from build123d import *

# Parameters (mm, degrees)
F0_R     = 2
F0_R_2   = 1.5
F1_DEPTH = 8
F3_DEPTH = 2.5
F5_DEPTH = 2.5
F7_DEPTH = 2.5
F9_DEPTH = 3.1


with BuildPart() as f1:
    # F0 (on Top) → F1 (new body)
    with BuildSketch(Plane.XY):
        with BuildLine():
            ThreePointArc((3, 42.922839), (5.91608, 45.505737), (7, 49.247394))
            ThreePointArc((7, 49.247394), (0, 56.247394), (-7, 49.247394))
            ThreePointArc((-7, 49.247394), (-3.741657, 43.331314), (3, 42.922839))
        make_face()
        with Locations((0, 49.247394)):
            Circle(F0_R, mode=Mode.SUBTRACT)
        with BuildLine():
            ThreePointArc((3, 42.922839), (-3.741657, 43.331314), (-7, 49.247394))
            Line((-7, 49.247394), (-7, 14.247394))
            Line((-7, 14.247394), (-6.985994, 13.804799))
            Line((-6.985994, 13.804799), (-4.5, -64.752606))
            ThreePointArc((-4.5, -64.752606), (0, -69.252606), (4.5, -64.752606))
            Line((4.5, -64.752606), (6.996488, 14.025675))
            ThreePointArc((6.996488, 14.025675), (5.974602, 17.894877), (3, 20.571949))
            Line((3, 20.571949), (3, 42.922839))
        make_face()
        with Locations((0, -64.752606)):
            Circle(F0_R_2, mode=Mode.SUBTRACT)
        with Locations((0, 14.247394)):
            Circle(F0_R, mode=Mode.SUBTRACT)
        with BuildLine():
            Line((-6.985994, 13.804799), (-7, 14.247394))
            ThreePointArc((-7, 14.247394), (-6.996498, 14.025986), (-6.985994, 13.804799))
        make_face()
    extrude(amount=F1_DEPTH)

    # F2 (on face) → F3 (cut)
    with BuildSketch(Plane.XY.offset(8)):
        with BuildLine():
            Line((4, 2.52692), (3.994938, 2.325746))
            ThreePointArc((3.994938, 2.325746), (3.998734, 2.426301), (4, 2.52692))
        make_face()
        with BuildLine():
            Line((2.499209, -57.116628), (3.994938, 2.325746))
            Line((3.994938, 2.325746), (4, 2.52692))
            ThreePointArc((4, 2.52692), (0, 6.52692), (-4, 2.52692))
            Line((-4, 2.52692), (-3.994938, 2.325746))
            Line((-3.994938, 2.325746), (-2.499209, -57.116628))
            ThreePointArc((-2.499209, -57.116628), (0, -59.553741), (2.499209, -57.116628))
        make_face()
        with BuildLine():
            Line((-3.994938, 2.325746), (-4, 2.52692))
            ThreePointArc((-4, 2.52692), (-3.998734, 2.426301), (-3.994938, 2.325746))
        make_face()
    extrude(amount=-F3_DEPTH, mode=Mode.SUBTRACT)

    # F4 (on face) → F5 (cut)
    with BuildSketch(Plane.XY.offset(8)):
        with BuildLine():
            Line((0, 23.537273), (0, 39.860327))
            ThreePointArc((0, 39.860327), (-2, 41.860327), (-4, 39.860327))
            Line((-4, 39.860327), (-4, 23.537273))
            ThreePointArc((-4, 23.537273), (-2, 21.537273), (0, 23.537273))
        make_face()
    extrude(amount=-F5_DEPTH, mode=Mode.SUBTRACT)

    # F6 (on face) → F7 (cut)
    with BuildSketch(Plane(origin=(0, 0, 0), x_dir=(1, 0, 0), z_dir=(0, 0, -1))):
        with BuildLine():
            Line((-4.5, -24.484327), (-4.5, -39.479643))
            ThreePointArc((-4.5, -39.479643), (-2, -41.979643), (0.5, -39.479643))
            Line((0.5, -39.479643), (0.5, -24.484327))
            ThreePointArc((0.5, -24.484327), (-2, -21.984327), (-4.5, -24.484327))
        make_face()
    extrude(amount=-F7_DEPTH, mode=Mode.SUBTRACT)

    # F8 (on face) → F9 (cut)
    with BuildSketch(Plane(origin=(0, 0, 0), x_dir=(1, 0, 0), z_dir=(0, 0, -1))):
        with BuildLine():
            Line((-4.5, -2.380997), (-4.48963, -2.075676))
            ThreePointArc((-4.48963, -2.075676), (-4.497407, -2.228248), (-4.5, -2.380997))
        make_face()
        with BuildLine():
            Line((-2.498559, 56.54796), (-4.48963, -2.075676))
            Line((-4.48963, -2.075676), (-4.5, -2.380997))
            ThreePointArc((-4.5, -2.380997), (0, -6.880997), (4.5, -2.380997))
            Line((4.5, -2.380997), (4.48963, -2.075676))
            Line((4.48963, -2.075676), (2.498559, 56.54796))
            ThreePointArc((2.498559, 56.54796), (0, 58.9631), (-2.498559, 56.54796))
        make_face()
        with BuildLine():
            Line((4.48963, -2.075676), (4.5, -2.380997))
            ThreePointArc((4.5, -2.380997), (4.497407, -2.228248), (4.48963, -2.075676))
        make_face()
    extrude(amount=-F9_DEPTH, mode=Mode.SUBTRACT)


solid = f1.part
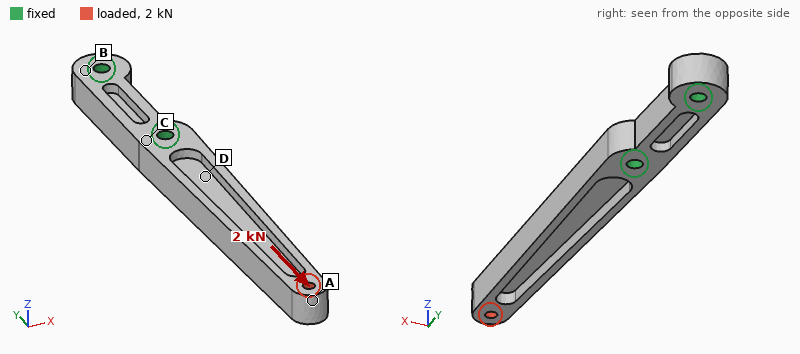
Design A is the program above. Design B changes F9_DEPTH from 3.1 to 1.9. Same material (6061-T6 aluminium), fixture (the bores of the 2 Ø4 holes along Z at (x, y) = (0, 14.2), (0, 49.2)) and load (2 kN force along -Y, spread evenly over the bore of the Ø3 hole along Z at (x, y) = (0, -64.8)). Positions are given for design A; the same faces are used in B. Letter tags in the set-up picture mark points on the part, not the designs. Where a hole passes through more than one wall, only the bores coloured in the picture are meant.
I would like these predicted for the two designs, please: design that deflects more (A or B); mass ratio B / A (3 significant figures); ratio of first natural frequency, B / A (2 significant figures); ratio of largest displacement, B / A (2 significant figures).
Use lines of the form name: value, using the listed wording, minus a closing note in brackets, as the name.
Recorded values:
design that deflects more: A
mass ratio B / A: 1.07
ratio of first natural frequency, B / A: 1.0
ratio of largest displacement, B / A: 0.52
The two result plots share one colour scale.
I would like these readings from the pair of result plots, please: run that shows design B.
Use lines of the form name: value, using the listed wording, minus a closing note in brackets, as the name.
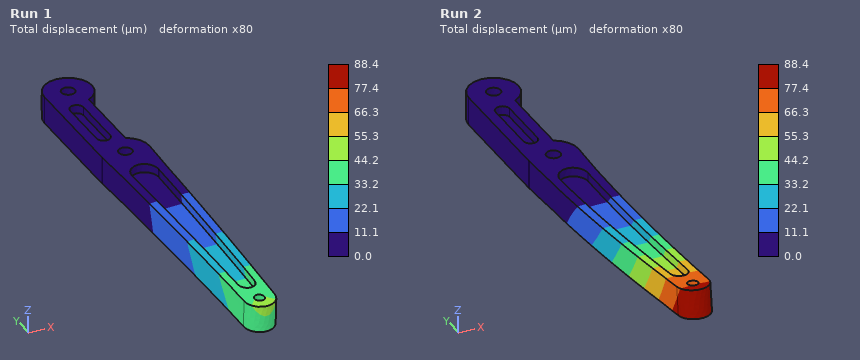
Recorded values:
run that shows design B: Run 1
